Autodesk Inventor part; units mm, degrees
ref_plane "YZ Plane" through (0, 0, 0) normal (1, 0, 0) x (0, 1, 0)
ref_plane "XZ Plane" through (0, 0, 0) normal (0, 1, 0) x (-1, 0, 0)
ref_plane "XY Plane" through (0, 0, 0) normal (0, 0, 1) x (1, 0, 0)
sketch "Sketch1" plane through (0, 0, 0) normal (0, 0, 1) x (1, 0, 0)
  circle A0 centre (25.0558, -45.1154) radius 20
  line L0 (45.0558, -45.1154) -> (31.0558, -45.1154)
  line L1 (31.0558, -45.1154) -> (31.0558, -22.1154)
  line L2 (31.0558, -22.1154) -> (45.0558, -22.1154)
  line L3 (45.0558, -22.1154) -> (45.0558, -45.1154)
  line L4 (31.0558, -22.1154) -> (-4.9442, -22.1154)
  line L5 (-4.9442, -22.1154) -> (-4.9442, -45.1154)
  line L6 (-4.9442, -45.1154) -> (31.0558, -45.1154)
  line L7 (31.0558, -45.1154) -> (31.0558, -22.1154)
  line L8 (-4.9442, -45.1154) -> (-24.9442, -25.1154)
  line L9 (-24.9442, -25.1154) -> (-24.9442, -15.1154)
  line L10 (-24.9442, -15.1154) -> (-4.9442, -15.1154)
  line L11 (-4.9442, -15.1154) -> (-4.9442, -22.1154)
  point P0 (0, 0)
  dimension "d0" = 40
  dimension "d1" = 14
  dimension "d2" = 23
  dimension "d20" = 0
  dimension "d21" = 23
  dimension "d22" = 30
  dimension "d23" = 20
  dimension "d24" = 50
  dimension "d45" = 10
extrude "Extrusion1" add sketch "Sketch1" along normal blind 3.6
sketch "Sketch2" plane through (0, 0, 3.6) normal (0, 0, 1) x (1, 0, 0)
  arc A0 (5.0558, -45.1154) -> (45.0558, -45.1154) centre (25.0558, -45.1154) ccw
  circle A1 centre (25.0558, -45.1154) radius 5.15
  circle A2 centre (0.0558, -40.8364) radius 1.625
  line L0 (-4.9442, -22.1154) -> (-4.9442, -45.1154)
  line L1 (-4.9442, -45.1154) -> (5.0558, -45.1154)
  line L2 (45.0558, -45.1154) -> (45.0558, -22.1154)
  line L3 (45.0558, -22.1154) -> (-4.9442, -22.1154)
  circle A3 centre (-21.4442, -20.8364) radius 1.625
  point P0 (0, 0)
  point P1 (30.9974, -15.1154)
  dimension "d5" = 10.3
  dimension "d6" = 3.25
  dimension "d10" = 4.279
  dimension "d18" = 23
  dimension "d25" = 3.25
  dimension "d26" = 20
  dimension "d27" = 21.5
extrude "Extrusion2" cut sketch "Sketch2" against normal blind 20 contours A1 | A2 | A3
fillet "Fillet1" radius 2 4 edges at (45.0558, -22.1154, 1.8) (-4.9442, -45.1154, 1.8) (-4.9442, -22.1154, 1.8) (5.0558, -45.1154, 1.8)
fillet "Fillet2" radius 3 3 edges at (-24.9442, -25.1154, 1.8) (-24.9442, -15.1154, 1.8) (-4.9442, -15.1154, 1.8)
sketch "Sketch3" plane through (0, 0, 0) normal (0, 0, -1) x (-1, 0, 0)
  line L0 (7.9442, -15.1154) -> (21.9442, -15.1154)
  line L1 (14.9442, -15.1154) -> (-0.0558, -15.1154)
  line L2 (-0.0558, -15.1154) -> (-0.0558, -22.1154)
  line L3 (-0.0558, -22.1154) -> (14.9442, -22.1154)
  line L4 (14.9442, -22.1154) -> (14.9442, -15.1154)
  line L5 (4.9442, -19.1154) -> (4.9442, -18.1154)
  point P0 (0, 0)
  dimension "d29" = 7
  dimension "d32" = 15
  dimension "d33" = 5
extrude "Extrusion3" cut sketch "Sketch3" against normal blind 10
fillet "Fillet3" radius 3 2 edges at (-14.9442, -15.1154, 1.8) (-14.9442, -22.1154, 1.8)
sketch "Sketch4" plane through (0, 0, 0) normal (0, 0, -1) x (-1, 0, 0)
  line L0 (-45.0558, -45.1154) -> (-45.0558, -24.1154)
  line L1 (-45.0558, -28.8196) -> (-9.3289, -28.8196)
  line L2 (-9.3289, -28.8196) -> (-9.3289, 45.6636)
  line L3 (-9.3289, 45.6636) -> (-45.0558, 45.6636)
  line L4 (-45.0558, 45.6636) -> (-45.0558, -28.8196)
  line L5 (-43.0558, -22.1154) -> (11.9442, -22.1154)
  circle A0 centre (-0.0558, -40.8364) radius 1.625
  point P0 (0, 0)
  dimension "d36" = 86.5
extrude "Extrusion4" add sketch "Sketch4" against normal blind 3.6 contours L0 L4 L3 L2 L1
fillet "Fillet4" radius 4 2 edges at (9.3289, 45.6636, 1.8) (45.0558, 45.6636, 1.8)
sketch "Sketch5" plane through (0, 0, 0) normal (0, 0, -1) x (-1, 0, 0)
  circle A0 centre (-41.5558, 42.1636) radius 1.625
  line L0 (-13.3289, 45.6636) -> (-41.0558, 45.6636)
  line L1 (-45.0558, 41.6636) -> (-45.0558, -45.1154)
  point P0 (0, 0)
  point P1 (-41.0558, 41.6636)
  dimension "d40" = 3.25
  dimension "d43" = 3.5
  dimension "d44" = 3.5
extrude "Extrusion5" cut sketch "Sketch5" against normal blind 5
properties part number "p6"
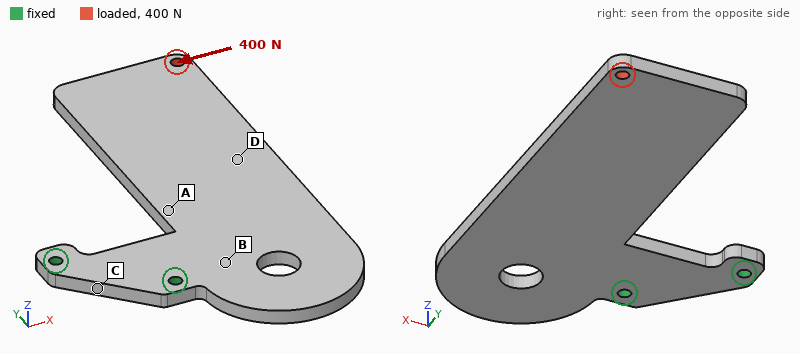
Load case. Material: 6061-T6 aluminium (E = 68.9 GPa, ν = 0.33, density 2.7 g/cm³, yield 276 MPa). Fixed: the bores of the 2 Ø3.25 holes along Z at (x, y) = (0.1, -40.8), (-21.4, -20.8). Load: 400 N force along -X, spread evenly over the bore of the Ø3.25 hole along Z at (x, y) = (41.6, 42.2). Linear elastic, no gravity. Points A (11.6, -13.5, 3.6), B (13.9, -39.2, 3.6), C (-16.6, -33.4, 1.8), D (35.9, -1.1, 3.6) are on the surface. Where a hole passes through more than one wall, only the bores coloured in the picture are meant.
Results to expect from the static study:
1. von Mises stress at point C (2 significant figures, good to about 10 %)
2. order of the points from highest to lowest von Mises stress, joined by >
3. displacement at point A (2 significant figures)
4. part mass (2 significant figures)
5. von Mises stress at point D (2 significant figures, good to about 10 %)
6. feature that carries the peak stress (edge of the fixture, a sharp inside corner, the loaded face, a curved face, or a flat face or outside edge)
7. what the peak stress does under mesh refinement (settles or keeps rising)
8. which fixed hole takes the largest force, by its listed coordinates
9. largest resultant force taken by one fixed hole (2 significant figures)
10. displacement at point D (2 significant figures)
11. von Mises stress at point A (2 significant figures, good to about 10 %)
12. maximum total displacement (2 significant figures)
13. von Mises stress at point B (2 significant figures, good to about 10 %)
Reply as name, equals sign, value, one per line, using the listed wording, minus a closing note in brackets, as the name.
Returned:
von Mises stress at point C = 61 MPa
order of the points from highest to lowest von Mises stress, joined by > = C > B > A > D
displacement at point A = 0.088 mm
part mass = 43 g
von Mises stress at point D = 13 MPa
feature that carries the peak stress = edge of the fixture
what the peak stress does under mesh refinement = keeps rising
which fixed hole takes the largest force, by its listed coordinates = (-21.4, -20.8)
largest resultant force taken by one fixed hole = 1.3 kN
displacement at point D = 0.19 mm
von Mises stress at point A = 26 MPa
maximum total displacement = 0.39 mm
von Mises stress at point B = 44 MPa
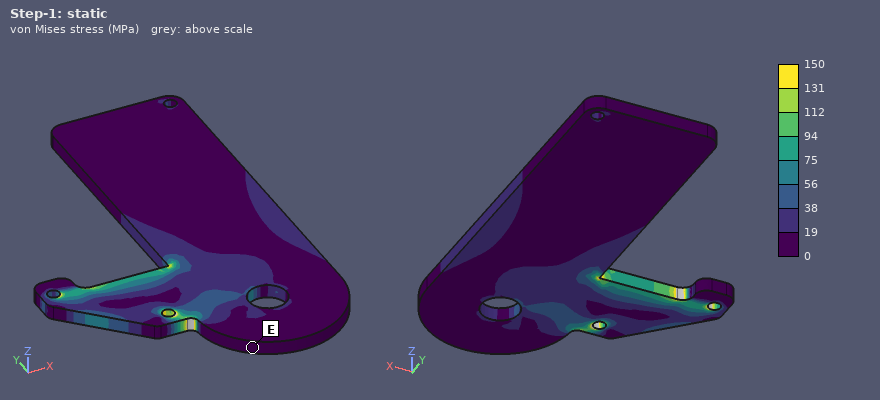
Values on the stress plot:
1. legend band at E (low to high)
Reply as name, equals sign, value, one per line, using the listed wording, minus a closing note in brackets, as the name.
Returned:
legend band at E = 0 to 19 MPa
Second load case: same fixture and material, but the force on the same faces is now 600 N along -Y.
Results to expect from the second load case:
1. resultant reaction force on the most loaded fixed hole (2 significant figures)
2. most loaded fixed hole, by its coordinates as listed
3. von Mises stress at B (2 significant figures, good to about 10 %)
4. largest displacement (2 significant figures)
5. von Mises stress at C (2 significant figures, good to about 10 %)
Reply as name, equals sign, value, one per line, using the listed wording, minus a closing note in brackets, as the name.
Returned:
resultant reaction force on the most loaded fixed hole = 1.2 kN
most loaded fixed hole, by its coordinates as listed = (0.1, -40.8)
von Mises stress at B = 32 MPa
largest displacement = 0.27 mm
von Mises stress at C = 44 MPa
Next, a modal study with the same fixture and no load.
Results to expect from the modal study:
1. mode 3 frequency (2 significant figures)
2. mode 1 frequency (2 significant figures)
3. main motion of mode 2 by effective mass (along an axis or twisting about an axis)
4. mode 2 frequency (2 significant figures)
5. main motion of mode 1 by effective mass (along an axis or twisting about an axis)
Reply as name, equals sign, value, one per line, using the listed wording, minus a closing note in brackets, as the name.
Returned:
mode 3 frequency = 1500 Hz
mode 1 frequency = 310 Hz
main motion of mode 2 by effective mass = along Z
mode 2 frequency = 930 Hz
main motion of mode 1 by effective mass = along Z
